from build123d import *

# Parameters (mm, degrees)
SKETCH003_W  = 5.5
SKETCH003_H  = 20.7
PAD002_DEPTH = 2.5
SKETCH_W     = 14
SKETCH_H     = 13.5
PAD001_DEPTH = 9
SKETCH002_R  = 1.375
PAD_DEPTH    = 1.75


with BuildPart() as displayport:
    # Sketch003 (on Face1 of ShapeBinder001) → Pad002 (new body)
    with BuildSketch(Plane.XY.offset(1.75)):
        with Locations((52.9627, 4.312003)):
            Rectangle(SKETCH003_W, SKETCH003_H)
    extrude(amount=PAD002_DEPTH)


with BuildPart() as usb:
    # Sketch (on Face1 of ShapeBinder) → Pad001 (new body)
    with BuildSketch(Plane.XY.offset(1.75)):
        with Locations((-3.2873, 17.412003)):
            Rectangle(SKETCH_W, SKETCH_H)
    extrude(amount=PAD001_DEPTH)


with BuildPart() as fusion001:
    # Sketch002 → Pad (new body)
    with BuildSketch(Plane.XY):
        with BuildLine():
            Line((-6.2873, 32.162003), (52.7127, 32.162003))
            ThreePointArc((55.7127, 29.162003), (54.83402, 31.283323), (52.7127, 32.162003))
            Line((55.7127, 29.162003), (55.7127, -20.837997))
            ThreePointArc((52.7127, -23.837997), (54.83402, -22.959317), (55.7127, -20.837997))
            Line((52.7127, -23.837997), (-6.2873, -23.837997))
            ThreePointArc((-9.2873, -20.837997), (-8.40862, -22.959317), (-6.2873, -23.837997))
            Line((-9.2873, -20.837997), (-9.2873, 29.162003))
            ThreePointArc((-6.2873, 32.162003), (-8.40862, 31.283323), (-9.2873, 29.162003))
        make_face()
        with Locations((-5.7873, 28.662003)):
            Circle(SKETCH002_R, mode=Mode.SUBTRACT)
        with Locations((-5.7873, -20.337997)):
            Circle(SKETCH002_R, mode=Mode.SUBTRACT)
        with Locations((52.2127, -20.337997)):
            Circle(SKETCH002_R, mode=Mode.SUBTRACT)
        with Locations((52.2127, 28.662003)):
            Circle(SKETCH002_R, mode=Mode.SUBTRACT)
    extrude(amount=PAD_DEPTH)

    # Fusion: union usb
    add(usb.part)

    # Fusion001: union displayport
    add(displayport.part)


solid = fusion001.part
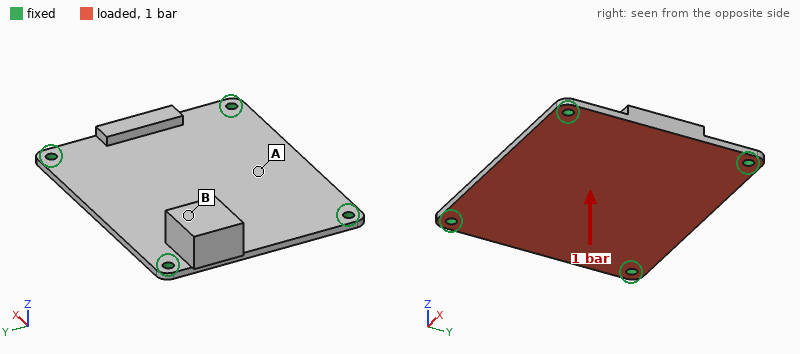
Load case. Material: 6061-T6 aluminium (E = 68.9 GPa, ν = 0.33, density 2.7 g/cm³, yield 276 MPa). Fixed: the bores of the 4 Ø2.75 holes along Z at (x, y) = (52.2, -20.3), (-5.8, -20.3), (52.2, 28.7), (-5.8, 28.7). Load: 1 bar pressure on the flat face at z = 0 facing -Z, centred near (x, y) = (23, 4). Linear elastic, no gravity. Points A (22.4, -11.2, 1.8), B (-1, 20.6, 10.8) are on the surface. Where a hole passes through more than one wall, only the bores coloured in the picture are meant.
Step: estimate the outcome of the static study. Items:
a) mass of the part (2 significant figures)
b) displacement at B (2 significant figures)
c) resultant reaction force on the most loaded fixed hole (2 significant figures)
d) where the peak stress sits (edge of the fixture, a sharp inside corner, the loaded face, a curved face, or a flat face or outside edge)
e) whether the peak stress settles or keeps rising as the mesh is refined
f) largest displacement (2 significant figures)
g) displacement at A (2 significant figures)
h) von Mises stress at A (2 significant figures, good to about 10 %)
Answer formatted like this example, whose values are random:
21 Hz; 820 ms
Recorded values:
22 g; 0.077 mm; 95 N; edge of the fixture; keeps rising; 0.18 mm; 0.16 mm; 32 MPa
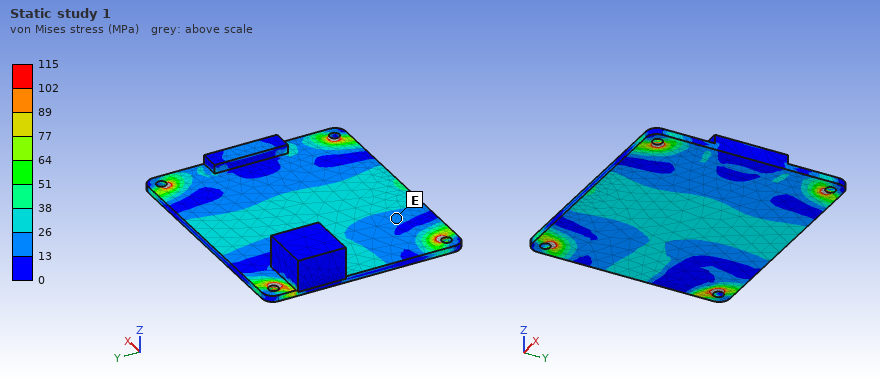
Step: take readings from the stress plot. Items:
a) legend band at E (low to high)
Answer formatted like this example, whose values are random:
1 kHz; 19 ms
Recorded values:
13 to 26 MPa
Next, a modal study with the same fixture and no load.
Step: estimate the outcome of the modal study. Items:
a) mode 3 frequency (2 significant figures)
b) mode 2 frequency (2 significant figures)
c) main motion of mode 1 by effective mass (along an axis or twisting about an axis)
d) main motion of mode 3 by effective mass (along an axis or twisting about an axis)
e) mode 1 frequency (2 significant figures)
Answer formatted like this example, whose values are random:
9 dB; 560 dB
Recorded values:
3400 Hz; 3200 Hz; along Z; twisting about X; 2000 Hz
